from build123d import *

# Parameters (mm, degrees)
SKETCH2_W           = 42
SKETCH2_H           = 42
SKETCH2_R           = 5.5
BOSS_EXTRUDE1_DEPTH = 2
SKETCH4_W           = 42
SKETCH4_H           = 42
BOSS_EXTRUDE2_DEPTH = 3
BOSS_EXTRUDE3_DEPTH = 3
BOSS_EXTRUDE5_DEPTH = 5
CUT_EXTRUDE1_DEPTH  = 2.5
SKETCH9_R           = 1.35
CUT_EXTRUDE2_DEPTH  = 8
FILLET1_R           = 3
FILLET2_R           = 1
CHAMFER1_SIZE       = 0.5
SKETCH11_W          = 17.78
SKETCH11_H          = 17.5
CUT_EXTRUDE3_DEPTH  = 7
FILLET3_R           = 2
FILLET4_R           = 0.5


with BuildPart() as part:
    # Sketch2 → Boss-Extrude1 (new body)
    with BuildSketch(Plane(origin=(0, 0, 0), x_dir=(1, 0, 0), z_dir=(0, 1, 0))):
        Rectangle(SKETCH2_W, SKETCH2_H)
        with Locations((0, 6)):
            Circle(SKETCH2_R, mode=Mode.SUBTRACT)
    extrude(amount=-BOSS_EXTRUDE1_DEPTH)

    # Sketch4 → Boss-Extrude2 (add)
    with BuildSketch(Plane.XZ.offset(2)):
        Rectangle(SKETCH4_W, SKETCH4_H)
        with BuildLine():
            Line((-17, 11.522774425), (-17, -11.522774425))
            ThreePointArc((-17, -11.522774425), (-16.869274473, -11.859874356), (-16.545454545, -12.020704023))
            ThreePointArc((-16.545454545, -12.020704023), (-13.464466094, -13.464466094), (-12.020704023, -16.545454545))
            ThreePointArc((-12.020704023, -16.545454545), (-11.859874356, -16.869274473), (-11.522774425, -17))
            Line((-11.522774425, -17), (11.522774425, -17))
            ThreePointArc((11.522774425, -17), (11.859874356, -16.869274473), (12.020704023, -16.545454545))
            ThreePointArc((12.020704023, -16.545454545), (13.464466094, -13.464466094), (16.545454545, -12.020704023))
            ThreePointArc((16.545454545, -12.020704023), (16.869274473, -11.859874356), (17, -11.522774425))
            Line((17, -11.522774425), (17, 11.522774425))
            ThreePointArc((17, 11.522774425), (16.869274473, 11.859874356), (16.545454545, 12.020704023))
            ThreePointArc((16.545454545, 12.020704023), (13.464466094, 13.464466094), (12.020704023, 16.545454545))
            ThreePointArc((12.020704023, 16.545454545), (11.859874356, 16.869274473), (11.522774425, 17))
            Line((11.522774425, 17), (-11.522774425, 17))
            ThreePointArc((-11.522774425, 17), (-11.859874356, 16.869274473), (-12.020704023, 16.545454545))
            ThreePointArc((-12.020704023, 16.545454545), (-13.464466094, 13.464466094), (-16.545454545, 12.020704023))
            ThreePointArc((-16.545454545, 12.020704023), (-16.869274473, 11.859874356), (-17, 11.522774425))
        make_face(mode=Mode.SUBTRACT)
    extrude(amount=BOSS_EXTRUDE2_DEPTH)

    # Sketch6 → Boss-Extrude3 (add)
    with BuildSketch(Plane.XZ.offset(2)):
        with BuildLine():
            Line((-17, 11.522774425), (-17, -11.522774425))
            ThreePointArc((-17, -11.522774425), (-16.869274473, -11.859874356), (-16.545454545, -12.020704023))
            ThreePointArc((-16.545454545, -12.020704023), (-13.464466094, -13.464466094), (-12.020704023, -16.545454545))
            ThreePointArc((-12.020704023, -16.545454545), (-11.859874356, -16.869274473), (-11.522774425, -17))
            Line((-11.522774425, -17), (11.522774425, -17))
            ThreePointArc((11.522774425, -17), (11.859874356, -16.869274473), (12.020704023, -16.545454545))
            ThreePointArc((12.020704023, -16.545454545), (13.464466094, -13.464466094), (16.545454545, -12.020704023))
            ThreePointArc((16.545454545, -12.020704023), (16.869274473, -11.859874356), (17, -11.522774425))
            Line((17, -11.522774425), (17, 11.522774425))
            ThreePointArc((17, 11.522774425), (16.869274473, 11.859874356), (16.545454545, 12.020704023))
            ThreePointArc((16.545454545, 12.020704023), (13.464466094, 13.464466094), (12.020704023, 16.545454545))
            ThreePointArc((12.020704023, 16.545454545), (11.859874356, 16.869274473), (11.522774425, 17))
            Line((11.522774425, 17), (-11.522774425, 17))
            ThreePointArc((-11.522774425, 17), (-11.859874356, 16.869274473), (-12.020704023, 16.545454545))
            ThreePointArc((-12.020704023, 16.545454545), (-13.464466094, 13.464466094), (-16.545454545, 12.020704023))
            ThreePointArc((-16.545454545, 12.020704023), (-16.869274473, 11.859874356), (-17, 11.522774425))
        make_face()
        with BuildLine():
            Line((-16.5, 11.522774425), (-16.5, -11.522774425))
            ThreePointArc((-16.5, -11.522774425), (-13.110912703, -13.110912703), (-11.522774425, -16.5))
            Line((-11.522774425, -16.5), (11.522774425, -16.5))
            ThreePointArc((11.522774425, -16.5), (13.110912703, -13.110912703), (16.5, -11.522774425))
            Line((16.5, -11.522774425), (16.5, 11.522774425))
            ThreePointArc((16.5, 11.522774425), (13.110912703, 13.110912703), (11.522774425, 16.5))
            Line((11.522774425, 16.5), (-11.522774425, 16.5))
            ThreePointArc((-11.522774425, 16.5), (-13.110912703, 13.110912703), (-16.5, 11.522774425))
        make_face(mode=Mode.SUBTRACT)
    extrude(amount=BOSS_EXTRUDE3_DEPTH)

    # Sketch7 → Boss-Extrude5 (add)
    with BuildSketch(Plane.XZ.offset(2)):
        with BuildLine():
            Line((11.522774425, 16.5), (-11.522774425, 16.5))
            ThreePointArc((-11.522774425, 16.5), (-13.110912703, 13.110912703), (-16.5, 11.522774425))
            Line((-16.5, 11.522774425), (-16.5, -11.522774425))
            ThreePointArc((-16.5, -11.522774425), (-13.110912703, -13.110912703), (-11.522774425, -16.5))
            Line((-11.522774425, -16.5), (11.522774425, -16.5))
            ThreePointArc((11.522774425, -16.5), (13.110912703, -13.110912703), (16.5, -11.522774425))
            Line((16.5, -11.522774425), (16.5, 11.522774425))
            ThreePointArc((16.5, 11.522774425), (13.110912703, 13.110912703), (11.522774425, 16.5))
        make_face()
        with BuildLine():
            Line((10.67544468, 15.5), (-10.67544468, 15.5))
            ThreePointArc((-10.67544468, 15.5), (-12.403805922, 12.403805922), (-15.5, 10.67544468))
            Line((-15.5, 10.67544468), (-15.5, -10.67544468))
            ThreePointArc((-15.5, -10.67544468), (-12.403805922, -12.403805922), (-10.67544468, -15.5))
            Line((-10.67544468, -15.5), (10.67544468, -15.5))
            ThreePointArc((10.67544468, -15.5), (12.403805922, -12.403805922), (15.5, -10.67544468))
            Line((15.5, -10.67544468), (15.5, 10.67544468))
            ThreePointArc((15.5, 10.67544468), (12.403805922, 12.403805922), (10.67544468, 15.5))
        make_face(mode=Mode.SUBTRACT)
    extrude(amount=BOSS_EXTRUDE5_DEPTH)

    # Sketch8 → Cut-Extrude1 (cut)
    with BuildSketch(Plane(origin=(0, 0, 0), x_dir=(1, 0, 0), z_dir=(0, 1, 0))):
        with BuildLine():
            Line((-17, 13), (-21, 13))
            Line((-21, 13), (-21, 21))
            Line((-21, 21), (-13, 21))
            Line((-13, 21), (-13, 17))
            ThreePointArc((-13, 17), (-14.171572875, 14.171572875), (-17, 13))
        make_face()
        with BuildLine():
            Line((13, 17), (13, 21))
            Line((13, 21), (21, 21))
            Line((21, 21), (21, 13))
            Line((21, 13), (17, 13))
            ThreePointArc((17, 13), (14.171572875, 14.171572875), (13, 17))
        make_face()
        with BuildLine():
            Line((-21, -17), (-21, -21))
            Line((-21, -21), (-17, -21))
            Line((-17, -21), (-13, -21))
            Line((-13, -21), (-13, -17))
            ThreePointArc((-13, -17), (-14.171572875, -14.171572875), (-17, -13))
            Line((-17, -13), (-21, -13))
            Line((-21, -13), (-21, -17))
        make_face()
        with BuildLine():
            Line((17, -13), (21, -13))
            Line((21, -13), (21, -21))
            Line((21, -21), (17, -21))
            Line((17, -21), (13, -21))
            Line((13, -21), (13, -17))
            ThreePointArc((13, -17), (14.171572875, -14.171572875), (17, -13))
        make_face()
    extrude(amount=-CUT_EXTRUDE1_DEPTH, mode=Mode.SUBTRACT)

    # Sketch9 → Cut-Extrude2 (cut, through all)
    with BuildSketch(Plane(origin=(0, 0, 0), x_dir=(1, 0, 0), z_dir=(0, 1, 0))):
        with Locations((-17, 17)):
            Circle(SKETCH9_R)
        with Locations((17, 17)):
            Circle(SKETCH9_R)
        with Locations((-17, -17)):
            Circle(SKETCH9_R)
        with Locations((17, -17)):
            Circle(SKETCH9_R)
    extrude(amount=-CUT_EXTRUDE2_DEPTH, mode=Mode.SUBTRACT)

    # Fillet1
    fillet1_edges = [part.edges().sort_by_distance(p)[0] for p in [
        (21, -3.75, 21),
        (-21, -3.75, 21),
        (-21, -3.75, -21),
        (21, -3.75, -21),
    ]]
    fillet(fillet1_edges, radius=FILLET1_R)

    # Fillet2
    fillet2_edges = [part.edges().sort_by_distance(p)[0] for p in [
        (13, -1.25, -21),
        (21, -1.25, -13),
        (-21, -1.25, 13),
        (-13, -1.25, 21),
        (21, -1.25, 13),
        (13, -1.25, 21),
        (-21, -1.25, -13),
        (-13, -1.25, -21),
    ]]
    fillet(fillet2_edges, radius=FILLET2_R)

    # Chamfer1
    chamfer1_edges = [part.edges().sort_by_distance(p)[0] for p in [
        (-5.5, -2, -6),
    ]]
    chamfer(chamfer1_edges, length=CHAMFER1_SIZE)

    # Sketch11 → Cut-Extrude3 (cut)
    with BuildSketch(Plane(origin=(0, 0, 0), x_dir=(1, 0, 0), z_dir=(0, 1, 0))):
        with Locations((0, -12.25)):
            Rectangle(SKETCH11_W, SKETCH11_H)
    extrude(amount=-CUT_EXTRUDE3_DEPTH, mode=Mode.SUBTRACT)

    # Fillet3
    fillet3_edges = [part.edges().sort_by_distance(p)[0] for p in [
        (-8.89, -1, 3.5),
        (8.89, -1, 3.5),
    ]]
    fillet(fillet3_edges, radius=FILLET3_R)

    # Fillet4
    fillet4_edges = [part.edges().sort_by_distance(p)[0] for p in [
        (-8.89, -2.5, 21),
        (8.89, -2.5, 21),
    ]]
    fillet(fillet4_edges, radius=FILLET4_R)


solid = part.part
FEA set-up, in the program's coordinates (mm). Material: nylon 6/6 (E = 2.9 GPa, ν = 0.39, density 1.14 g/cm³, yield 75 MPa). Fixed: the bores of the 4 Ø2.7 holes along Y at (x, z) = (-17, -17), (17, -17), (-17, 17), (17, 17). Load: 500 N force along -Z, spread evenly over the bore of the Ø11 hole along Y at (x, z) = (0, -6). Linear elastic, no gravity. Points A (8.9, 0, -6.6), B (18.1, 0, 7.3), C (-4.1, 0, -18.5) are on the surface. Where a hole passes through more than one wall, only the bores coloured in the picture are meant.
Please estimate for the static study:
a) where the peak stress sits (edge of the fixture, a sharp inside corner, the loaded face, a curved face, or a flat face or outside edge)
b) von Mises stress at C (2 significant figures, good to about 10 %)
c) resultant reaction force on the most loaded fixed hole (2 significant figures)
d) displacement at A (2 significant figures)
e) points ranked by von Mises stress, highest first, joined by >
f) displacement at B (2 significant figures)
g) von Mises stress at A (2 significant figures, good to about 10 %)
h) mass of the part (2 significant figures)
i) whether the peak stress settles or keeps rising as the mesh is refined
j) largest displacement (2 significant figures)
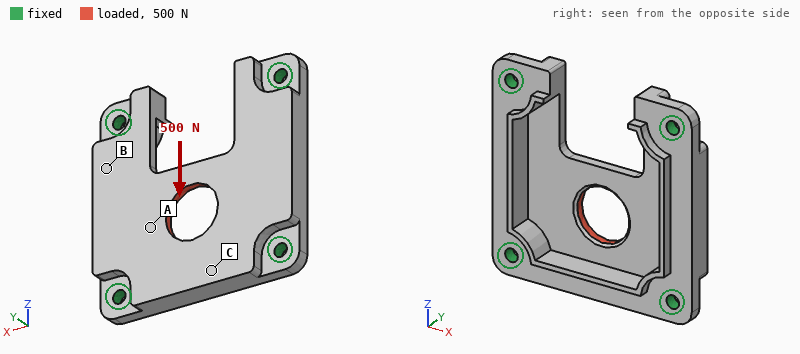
edge of the fixture
6.6 MPa
140 N
0.086 mm
A > C > B
0.033 mm
10 MPa
5.2 g
keeps rising
0.15 mm
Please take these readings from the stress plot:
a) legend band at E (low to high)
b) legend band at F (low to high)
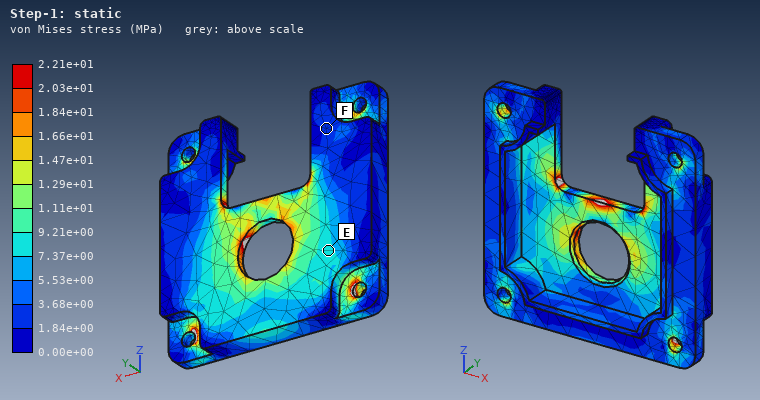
7.37e+00 to 9.21e+00 MPa
1.84e+00 to 3.68e+00 MPa
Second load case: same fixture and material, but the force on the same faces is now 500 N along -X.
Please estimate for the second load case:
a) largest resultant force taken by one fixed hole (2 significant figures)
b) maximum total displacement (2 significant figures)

210 N
0.10 mm
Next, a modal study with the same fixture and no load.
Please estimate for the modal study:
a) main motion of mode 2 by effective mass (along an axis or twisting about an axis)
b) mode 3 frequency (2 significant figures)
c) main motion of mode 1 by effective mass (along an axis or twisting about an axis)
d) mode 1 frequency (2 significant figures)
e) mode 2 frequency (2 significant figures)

twisting about Z
5200 Hz
along Y
3500 Hz
4900 Hz
